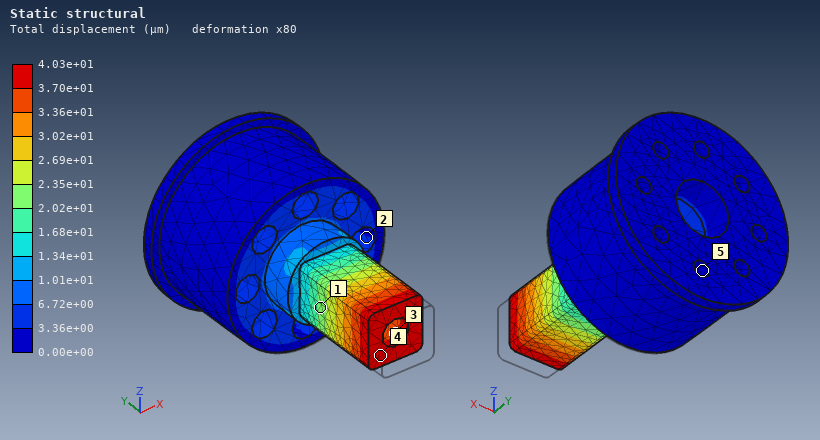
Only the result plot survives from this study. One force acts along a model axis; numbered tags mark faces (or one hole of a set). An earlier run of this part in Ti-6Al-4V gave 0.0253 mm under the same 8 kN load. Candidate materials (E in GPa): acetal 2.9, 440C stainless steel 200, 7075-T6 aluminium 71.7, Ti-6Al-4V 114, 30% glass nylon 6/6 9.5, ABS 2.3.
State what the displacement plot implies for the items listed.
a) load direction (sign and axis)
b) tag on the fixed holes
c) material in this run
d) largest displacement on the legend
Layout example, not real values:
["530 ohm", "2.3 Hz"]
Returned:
["+Y", "5", "7075-T6 aluminium", "4.03e+01 µm"]
